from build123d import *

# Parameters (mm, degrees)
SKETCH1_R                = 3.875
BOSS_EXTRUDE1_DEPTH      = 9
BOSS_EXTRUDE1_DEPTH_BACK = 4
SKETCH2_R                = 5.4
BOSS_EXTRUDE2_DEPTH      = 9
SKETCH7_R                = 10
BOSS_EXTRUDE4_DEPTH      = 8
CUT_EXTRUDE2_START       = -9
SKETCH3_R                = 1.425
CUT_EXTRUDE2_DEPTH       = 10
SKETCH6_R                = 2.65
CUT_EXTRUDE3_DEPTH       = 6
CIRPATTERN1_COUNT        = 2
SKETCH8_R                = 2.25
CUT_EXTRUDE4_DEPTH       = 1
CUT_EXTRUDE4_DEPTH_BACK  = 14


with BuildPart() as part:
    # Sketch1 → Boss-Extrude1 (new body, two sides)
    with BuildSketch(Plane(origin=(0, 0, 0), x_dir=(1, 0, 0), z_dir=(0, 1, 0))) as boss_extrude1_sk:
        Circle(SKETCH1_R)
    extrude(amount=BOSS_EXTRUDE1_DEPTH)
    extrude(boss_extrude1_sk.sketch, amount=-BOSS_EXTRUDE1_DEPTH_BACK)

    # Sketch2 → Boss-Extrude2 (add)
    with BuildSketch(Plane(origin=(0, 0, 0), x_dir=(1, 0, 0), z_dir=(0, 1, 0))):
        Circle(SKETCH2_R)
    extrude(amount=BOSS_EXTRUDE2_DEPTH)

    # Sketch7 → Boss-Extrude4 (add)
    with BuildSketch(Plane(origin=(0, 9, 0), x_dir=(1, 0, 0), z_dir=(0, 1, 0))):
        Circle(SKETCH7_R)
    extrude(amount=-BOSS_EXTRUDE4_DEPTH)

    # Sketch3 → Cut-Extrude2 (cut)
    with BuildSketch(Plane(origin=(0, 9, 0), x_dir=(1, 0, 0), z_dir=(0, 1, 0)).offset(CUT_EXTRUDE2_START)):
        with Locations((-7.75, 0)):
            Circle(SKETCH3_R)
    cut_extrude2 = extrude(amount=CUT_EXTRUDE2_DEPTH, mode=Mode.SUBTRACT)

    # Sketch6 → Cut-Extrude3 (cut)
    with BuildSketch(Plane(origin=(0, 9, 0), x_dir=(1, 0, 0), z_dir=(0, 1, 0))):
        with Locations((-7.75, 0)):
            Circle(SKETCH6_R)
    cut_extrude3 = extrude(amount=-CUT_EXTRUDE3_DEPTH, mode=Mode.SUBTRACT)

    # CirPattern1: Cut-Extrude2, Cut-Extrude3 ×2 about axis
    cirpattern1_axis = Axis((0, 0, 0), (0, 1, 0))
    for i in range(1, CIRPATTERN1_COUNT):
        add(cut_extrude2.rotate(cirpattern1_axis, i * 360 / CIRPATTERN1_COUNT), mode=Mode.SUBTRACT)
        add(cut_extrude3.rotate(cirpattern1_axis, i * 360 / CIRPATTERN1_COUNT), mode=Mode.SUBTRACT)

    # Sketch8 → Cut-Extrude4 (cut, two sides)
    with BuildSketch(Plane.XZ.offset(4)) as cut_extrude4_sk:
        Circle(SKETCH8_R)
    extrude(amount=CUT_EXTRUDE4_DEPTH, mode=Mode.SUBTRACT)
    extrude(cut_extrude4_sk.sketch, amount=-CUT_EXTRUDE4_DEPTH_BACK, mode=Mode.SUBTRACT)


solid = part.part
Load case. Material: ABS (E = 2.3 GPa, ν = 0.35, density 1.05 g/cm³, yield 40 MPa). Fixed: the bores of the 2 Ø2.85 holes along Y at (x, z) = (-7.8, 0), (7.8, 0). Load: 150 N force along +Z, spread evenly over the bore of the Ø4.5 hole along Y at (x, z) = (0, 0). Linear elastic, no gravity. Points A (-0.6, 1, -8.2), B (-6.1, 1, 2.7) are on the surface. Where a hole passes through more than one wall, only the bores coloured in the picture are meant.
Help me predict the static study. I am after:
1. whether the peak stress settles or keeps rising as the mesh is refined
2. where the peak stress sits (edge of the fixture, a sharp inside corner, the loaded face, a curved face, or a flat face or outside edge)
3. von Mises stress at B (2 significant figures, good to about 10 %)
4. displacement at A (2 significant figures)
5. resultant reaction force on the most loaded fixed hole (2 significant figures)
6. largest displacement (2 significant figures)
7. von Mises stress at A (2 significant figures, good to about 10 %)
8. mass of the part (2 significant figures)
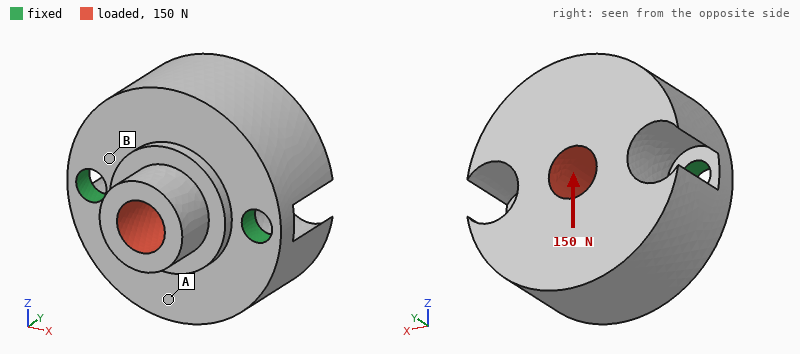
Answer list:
keeps rising
edge of the fixture
3.3 MPa
23 µm
75 N
41 µm
1.2 MPa
2.4 g
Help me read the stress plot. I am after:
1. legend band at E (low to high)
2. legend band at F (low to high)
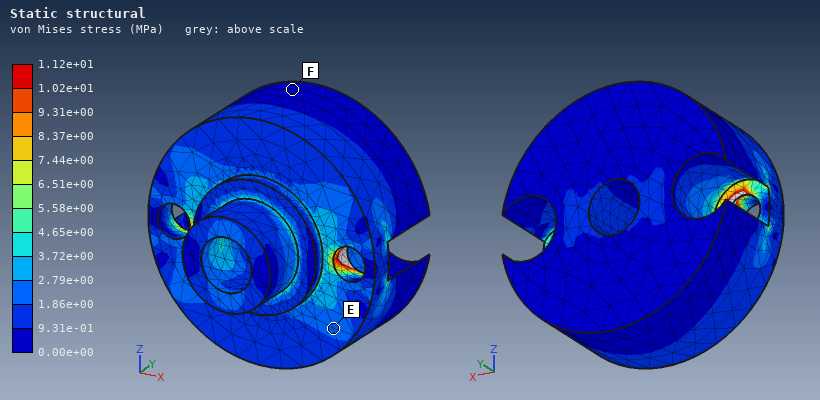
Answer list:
1.86e+00 to 2.79e+00 MPa
0.00e+00 to 9.31e-01 MPa
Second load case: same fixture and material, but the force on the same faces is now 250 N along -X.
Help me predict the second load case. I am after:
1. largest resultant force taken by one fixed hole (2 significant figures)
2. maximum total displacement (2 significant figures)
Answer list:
130 N
32 µm
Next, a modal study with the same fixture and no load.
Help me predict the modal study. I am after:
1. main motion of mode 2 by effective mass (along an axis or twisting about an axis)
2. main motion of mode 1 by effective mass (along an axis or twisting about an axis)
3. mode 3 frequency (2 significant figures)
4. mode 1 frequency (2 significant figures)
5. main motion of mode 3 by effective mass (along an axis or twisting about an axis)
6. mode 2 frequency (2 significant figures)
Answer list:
along Y
along Z
12 kHz
3200 Hz
along X
9500 Hz
